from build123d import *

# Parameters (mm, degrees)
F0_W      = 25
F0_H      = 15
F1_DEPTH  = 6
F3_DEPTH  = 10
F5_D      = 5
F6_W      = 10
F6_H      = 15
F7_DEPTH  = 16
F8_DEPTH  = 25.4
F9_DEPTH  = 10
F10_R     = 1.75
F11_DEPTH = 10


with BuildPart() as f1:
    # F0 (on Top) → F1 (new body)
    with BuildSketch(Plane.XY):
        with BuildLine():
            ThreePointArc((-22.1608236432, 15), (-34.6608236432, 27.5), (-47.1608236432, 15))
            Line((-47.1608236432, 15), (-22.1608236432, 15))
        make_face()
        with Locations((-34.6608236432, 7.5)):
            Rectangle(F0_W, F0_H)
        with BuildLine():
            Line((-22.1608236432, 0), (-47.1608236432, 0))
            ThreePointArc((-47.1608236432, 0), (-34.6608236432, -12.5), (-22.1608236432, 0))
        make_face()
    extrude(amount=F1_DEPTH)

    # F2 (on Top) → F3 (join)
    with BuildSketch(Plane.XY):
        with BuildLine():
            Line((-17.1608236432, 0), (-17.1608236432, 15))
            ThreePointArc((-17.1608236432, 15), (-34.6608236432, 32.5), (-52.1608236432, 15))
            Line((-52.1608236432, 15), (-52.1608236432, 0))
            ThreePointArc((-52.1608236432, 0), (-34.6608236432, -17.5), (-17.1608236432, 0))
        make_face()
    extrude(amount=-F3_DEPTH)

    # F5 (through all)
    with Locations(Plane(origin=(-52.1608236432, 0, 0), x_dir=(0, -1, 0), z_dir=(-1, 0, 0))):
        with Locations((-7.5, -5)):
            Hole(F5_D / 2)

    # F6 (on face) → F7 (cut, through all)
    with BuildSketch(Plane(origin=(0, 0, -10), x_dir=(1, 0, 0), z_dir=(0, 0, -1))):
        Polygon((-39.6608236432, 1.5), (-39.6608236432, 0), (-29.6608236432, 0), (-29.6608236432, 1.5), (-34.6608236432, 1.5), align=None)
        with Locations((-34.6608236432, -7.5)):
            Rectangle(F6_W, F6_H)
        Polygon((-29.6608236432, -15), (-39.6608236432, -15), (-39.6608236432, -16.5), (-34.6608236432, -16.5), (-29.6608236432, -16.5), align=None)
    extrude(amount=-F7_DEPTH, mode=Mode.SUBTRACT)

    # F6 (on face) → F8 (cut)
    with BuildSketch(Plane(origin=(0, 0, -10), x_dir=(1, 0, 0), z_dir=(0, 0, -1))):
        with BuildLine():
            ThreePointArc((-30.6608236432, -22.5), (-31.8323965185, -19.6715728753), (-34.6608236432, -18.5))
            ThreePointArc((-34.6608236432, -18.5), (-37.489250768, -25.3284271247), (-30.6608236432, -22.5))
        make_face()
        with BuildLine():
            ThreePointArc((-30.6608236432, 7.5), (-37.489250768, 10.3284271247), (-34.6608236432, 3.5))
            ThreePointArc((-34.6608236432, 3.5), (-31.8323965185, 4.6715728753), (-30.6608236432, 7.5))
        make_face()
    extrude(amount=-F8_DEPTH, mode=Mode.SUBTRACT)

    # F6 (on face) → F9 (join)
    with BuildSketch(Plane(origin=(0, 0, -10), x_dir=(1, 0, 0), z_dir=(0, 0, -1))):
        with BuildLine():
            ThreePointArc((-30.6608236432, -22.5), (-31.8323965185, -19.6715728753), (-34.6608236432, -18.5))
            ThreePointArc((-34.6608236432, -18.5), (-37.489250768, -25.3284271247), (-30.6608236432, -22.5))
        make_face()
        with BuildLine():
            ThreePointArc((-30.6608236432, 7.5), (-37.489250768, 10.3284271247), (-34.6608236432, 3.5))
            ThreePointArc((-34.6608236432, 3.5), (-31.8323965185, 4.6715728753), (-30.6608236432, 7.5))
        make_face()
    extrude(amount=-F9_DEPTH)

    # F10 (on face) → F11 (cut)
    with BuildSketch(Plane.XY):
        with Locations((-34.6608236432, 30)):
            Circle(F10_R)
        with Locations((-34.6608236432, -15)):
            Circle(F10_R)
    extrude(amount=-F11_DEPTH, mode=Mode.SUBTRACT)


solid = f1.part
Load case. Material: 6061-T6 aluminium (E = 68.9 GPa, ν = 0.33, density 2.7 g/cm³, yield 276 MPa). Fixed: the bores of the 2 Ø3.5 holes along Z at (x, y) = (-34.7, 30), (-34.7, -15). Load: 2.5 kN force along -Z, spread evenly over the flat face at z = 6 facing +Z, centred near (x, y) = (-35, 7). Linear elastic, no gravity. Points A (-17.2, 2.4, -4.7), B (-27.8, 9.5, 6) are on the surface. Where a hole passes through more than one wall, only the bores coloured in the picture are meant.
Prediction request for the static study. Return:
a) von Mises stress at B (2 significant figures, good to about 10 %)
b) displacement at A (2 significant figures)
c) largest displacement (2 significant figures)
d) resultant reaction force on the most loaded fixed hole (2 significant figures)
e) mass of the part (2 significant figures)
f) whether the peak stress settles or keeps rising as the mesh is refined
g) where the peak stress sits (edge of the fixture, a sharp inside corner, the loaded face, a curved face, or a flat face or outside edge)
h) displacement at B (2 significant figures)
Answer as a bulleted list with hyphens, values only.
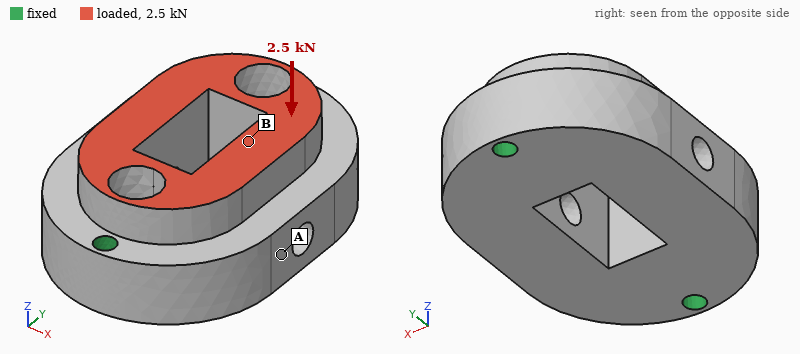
- 14 MPa
- 8.6 µm
- 9.0 µm
- 1.3 kN
- 43 g
- keeps rising
- edge of the fixture
- 7.9 µm
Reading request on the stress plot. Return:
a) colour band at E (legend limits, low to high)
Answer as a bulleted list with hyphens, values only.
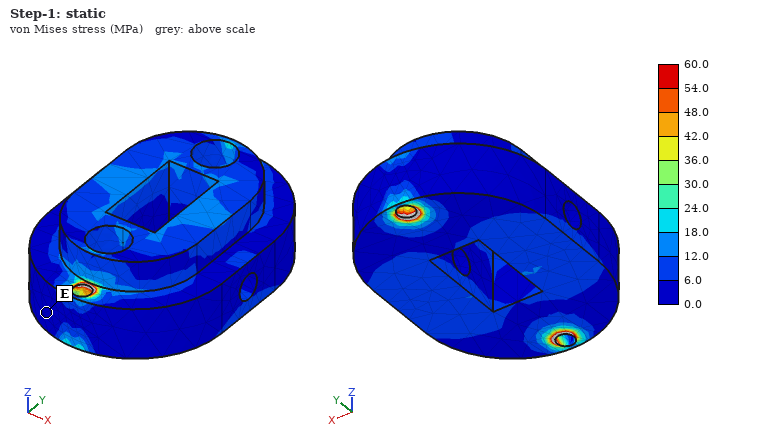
- 0.0 to 6.0 MPa
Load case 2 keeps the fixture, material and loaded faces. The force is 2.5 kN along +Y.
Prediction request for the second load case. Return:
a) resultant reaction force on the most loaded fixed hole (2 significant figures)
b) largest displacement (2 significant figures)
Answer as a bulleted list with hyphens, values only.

- 1.4 kN
- 6.1 µm
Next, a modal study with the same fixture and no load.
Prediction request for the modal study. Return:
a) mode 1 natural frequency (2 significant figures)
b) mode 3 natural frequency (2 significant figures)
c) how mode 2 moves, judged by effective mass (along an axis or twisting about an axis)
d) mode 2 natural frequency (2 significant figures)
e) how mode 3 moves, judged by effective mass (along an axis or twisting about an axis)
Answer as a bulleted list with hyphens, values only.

- 12 kHz
- 23 kHz
- along Z
- 15 kHz
- along X
